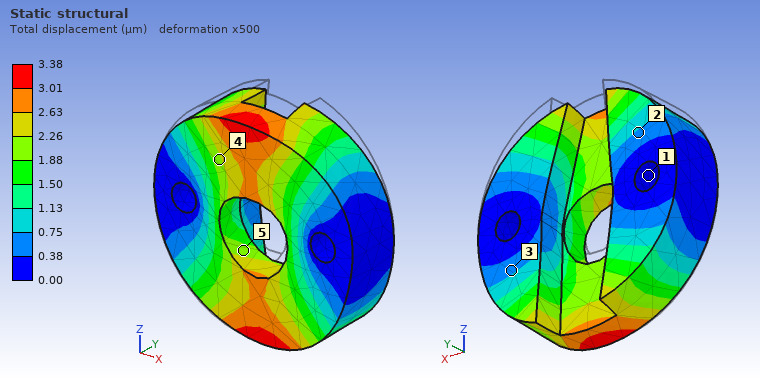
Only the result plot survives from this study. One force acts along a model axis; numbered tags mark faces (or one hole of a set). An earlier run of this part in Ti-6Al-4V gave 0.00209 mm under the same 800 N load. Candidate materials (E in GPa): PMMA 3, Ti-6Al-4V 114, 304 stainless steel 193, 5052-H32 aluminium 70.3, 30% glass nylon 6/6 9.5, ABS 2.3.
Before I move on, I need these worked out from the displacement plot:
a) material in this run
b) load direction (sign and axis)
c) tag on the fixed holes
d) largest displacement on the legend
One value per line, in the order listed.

5052-H32 aluminium
-Z
1
3.38 µm
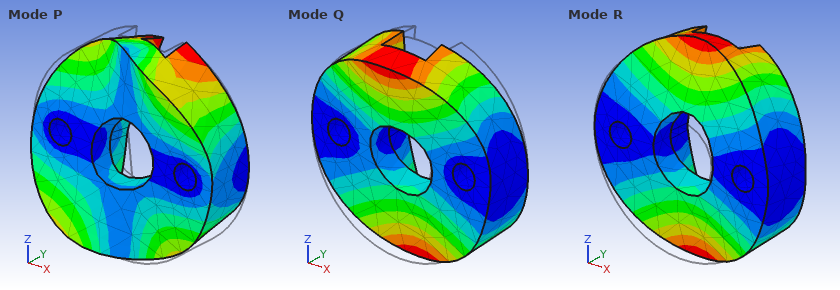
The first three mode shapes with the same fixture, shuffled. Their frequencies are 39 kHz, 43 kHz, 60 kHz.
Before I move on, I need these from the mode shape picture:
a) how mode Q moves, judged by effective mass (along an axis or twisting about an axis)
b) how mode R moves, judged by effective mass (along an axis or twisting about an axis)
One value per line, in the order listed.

twisting about X
along Y
